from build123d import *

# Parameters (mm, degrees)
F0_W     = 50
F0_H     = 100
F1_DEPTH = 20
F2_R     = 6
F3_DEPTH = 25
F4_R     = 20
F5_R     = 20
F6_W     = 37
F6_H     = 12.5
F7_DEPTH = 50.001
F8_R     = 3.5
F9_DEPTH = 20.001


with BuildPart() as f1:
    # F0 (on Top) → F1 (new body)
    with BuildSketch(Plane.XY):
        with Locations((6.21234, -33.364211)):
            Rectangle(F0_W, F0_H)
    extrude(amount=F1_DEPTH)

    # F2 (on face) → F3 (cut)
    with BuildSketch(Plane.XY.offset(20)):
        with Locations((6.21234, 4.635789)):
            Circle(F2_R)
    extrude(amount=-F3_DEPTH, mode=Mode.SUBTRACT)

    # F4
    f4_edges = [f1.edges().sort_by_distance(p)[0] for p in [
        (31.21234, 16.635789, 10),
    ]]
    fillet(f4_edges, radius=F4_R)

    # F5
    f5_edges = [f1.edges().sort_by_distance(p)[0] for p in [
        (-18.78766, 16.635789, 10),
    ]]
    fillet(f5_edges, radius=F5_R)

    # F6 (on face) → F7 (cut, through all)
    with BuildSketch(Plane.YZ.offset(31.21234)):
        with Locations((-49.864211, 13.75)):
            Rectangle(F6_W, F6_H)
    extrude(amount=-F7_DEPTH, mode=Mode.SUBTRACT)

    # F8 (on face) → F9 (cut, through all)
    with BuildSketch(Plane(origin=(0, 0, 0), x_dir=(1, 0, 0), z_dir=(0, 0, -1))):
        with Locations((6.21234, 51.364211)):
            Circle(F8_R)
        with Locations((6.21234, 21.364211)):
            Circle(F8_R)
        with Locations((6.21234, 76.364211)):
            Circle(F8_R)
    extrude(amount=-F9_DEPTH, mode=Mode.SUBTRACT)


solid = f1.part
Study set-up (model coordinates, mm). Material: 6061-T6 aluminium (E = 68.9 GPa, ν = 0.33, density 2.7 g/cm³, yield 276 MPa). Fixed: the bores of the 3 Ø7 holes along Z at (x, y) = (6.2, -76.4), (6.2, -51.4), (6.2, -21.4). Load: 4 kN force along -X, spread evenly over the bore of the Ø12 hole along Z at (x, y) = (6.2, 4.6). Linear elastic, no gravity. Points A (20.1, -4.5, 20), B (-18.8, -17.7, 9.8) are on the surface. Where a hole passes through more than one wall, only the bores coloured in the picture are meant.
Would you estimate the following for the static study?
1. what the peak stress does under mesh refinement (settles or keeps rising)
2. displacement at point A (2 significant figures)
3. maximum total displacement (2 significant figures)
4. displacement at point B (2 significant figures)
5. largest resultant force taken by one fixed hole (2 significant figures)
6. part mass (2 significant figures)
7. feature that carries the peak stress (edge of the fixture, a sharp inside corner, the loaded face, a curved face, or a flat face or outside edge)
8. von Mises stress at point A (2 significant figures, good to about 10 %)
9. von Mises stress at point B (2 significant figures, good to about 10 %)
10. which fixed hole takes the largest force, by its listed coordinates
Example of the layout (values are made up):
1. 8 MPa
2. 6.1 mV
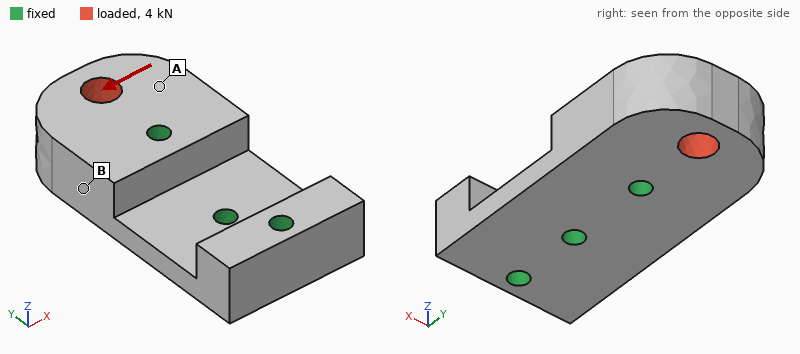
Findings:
1. keeps rising
2. 11 µm
3. 25 µm
4. 11 µm
5. 5.7 kN
6. 190 g
7. edge of the fixture
8. 5.8 MPa
9. 12 MPa
10. (6.2, -21.4)
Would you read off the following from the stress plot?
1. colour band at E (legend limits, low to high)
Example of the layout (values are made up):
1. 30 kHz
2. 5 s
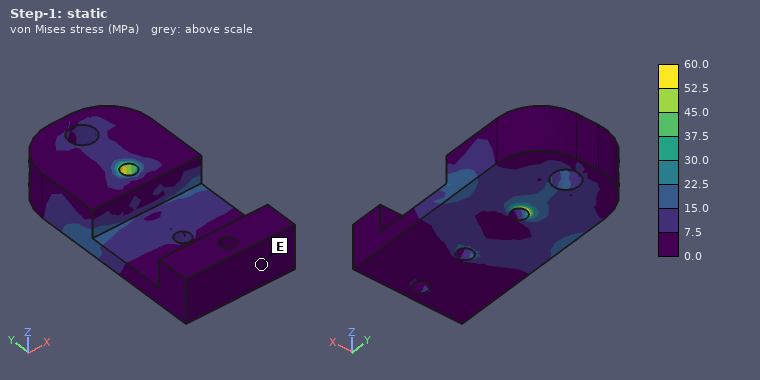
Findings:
1. 0.0 to 7.5 MPa
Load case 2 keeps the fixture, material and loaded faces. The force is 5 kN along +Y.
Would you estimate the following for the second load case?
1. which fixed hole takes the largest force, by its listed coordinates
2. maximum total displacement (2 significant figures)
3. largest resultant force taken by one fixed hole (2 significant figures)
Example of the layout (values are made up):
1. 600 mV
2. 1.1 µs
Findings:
1. (6.2, -21.4)
2. 6.8 µm
3. 4.3 kN
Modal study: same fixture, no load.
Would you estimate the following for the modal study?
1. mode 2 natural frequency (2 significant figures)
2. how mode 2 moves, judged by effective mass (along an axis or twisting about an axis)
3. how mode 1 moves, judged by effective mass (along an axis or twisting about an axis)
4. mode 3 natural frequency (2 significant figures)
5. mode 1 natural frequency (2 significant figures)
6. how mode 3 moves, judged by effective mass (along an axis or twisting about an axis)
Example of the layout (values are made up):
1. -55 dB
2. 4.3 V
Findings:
1. 9300 Hz
2. along X
3. along Z
4. 12 kHz
5. 8800 Hz
6. twisting about Y
